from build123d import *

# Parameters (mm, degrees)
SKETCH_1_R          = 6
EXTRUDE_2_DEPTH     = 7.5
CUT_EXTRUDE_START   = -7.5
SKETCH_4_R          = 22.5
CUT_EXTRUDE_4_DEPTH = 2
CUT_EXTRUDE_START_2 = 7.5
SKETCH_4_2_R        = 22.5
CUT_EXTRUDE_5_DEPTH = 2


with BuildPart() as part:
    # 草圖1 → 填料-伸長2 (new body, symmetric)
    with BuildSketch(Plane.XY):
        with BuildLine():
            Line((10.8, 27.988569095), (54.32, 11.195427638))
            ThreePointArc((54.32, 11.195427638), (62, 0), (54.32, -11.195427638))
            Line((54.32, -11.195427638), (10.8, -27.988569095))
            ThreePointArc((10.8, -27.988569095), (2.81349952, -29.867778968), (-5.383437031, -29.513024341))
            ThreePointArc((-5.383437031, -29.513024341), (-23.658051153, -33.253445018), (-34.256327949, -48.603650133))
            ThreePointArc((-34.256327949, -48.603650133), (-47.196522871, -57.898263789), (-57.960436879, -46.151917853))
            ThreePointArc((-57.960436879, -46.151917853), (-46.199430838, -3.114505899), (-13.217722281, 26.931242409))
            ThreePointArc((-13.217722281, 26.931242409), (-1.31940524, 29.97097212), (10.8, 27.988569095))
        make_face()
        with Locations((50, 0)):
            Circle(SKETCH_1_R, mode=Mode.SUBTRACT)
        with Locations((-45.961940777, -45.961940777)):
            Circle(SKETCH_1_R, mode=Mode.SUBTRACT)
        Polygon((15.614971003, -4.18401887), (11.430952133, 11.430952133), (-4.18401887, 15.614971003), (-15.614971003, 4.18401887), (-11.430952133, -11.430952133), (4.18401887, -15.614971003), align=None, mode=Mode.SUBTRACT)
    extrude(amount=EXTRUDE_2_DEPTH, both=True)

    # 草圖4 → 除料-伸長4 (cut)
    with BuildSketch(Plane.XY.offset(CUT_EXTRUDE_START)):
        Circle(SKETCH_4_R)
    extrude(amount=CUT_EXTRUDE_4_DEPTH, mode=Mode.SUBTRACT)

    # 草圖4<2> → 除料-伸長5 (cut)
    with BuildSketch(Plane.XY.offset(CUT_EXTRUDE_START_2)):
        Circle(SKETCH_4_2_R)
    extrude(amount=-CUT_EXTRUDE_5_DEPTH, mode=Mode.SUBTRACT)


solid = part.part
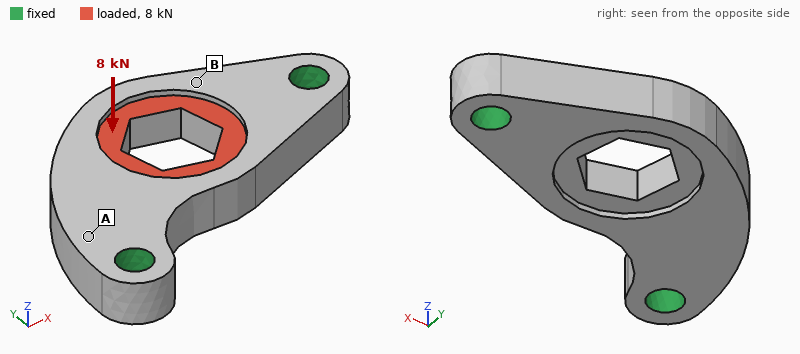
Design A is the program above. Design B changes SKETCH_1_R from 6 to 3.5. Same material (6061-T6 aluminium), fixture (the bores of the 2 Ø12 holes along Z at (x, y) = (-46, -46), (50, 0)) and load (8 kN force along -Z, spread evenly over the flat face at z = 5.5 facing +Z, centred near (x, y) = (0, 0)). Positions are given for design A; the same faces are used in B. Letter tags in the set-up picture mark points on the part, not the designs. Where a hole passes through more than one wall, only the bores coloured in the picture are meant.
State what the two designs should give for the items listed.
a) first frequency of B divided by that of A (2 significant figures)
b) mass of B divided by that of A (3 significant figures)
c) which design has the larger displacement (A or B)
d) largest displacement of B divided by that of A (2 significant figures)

0.89
1.03
B
1.2
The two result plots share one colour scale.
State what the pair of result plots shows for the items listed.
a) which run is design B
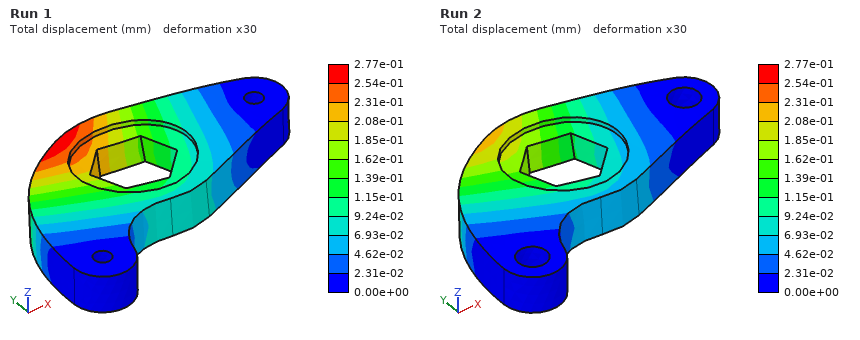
Run 1
